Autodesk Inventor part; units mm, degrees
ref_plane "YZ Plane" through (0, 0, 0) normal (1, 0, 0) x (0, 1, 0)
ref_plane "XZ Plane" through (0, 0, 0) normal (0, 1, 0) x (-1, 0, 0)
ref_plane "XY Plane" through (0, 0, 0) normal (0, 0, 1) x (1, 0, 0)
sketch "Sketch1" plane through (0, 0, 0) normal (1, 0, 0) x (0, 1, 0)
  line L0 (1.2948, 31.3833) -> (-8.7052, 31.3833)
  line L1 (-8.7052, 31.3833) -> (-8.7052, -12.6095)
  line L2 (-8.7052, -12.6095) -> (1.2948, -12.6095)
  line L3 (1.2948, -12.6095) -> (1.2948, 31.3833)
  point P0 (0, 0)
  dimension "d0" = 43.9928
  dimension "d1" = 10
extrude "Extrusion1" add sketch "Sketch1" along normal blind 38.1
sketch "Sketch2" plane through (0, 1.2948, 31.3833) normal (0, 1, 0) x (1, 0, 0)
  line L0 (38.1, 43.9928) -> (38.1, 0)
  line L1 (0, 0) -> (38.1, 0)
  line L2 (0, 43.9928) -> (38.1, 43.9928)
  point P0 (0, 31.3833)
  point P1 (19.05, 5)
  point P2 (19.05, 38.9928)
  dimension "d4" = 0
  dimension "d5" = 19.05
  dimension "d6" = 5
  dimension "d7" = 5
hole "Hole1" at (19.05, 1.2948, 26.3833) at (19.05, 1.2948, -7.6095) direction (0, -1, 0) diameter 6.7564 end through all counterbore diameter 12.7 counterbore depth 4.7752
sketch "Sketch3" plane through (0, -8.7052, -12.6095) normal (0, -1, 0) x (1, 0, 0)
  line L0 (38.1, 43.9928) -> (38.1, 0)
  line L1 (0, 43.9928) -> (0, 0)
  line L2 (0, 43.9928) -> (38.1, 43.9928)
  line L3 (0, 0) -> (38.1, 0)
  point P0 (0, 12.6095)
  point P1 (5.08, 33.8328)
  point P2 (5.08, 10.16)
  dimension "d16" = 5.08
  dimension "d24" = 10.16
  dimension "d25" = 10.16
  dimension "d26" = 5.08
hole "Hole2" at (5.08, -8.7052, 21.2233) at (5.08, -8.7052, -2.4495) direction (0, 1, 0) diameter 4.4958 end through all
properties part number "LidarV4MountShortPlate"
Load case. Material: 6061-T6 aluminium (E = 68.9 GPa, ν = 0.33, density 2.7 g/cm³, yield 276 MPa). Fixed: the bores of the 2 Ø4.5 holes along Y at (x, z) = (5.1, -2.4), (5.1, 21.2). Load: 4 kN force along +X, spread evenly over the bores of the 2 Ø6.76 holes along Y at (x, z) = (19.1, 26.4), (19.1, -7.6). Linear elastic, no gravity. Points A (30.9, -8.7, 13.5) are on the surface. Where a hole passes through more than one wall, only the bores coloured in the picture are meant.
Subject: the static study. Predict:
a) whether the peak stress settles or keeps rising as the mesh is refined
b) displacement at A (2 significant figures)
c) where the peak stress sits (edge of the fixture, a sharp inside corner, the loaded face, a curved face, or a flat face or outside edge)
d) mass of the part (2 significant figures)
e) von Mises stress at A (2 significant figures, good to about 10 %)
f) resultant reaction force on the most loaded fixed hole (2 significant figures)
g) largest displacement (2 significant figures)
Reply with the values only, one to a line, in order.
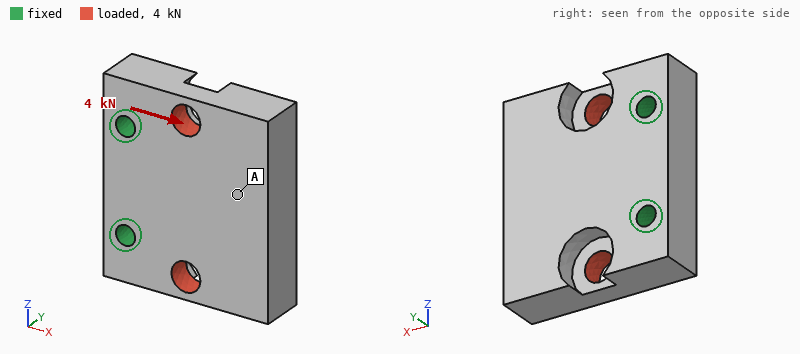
keeps rising
12 µm
edge of the fixture
40 g
5.7 MPa
2.0 kN
18 µm
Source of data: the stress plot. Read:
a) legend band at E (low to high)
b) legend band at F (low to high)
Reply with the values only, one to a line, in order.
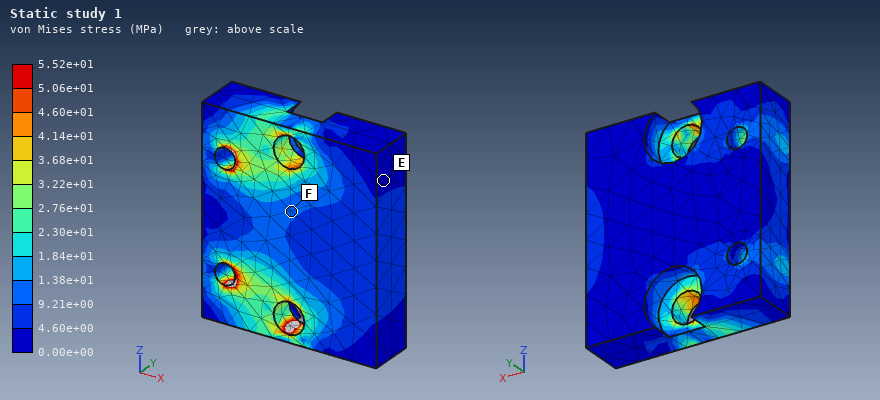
0.00e+00 to 4.60e+00 MPa
9.21e+00 to 1.38e+01 MPa
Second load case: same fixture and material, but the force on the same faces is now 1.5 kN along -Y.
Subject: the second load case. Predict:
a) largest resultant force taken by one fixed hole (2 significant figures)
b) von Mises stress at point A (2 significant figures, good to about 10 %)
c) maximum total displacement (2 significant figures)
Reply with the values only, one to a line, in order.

750 N
7.0 MPa
28 µm
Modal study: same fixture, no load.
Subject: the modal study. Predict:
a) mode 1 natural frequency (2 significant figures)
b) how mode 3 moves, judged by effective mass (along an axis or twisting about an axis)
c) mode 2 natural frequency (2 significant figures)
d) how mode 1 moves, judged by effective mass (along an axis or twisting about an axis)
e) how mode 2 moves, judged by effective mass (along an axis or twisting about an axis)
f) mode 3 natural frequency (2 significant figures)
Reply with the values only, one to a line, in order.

5700 Hz
along Z
10 kHz
along Y
twisting about X
14 kHz
